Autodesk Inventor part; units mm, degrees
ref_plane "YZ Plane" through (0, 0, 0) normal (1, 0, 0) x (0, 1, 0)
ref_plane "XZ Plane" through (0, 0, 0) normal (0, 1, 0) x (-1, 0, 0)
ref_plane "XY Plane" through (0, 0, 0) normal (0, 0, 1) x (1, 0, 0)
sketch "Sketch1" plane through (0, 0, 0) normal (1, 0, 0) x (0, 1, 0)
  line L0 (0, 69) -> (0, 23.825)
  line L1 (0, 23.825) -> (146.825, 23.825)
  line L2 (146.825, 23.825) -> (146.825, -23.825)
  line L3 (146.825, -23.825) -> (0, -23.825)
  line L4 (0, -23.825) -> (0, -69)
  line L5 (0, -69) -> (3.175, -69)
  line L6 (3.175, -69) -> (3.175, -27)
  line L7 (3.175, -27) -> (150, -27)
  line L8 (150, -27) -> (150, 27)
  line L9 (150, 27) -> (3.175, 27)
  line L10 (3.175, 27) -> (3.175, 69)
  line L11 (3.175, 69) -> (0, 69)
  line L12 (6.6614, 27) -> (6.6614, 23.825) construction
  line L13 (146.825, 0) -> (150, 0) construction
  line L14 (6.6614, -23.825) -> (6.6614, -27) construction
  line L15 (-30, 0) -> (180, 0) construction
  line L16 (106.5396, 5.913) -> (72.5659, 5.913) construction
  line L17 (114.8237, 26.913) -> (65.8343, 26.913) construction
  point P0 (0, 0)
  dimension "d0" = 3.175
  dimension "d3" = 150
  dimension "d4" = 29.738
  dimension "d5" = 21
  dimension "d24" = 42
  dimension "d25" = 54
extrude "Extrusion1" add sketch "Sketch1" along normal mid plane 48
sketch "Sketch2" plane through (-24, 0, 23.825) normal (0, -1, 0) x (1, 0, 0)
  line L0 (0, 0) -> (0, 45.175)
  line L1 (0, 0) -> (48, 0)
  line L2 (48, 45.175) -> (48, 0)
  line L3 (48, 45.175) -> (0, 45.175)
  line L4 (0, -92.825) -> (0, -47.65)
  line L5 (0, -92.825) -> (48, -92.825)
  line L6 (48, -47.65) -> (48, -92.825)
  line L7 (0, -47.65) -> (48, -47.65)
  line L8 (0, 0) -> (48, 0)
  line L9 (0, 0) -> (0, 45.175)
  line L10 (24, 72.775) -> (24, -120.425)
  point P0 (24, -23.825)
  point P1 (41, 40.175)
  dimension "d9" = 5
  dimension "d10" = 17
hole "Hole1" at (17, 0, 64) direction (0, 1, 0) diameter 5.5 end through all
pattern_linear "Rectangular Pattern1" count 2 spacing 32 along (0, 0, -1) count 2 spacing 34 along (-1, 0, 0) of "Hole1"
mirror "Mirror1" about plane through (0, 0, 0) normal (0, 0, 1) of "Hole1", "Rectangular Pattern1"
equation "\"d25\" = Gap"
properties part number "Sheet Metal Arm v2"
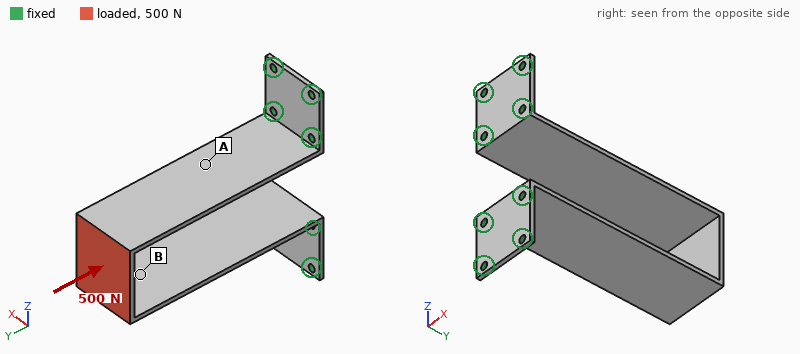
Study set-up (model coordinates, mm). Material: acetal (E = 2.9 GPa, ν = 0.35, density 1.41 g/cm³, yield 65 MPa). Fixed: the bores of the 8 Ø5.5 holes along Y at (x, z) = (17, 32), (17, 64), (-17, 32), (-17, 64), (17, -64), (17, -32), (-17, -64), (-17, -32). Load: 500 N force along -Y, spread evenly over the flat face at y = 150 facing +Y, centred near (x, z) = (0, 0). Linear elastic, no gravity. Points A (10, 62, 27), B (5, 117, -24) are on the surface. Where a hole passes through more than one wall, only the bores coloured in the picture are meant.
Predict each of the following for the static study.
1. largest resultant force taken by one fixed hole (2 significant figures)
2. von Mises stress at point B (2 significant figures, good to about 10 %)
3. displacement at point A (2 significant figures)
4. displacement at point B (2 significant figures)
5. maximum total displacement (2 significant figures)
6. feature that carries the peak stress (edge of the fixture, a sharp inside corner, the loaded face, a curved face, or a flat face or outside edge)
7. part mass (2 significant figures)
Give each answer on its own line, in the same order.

130 N
8.2 MPa
1.0 mm
1.5 mm
1.7 mm
the loaded face
92 g
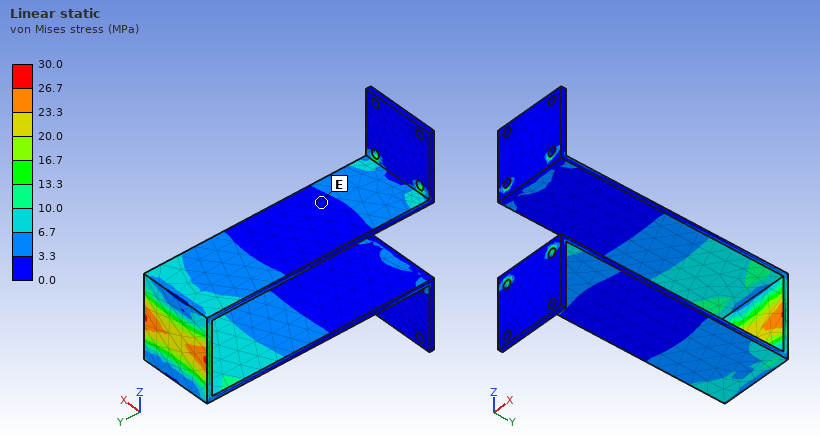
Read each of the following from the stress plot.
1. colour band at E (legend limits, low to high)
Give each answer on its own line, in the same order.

0.0 to 3.3 MPa
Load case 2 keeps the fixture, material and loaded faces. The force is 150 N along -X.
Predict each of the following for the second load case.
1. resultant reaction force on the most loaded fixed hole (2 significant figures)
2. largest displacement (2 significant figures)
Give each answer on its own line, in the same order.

320 N
2.0 mm
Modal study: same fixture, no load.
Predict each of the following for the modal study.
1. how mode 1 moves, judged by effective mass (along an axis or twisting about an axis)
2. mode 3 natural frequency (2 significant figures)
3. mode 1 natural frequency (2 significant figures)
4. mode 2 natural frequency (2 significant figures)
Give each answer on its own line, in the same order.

along Z
240 Hz
43 Hz
180 Hz
